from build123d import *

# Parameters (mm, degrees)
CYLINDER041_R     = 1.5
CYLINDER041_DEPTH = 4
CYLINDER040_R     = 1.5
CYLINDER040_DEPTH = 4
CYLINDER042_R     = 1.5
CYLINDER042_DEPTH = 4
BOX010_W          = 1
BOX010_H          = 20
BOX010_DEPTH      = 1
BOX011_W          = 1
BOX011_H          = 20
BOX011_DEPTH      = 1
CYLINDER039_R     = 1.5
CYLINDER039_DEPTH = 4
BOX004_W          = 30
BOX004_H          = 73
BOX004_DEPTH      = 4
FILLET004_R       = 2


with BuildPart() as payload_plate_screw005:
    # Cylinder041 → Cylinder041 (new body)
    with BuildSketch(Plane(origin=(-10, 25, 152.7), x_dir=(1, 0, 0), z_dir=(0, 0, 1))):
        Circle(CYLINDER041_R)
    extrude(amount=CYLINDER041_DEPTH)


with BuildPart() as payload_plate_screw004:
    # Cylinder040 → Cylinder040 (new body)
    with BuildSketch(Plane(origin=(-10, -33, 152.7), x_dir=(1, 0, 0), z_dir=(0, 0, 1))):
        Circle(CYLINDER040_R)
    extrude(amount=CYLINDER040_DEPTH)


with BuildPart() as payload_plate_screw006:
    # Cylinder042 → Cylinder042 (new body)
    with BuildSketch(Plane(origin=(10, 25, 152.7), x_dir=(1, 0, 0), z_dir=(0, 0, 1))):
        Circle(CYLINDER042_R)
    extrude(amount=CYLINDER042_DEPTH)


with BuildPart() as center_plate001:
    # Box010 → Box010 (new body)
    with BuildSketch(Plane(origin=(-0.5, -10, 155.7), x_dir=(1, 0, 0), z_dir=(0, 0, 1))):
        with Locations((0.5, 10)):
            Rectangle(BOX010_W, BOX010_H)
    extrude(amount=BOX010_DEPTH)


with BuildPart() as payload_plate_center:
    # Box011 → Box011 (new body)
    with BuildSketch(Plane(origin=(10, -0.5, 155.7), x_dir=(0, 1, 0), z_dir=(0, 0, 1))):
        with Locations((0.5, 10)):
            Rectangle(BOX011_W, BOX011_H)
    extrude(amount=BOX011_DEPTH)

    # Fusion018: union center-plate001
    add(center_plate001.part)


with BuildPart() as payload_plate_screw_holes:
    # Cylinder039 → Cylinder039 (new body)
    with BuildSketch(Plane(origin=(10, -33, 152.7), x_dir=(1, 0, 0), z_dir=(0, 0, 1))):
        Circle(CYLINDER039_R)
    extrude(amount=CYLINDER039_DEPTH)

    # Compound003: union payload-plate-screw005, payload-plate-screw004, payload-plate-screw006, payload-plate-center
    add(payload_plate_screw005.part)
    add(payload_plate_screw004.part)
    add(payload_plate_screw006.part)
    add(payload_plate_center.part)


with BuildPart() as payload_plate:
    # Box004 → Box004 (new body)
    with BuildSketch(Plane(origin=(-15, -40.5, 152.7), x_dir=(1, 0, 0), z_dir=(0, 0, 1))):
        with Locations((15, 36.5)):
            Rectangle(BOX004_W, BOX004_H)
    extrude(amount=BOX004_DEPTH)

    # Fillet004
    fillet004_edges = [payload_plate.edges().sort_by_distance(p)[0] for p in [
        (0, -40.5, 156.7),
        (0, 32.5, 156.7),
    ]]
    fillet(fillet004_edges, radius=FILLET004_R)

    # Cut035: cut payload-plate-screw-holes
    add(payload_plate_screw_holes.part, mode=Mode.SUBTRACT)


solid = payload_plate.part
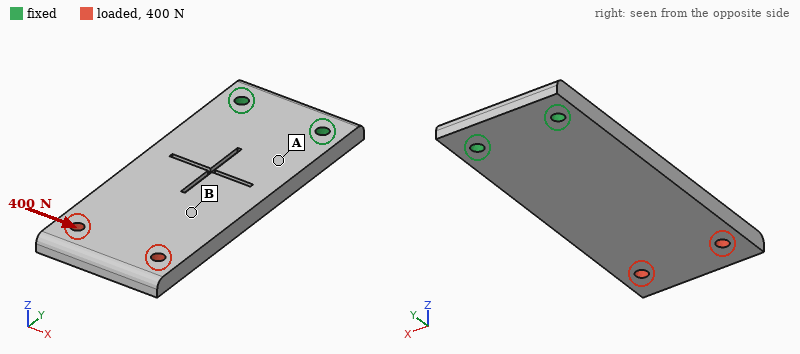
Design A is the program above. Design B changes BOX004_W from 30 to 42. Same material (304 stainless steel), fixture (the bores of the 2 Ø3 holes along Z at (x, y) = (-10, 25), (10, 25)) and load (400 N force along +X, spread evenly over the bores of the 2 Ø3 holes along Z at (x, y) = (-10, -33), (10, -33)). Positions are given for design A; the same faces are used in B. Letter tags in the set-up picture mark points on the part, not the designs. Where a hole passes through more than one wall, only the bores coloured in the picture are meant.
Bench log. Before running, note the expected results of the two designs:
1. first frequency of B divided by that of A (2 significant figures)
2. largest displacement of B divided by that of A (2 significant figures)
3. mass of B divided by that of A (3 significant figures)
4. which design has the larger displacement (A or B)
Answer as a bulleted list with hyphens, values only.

- 0.99
- 0.63
- 1.41
- A
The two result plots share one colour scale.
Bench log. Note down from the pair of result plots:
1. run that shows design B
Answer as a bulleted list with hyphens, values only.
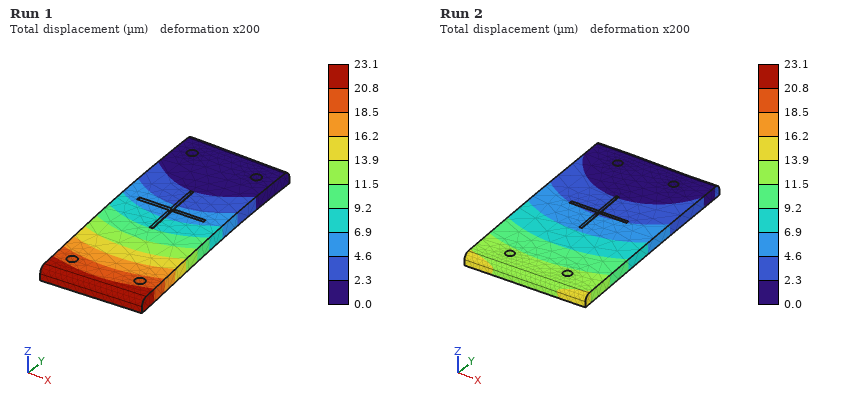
- Run 2
